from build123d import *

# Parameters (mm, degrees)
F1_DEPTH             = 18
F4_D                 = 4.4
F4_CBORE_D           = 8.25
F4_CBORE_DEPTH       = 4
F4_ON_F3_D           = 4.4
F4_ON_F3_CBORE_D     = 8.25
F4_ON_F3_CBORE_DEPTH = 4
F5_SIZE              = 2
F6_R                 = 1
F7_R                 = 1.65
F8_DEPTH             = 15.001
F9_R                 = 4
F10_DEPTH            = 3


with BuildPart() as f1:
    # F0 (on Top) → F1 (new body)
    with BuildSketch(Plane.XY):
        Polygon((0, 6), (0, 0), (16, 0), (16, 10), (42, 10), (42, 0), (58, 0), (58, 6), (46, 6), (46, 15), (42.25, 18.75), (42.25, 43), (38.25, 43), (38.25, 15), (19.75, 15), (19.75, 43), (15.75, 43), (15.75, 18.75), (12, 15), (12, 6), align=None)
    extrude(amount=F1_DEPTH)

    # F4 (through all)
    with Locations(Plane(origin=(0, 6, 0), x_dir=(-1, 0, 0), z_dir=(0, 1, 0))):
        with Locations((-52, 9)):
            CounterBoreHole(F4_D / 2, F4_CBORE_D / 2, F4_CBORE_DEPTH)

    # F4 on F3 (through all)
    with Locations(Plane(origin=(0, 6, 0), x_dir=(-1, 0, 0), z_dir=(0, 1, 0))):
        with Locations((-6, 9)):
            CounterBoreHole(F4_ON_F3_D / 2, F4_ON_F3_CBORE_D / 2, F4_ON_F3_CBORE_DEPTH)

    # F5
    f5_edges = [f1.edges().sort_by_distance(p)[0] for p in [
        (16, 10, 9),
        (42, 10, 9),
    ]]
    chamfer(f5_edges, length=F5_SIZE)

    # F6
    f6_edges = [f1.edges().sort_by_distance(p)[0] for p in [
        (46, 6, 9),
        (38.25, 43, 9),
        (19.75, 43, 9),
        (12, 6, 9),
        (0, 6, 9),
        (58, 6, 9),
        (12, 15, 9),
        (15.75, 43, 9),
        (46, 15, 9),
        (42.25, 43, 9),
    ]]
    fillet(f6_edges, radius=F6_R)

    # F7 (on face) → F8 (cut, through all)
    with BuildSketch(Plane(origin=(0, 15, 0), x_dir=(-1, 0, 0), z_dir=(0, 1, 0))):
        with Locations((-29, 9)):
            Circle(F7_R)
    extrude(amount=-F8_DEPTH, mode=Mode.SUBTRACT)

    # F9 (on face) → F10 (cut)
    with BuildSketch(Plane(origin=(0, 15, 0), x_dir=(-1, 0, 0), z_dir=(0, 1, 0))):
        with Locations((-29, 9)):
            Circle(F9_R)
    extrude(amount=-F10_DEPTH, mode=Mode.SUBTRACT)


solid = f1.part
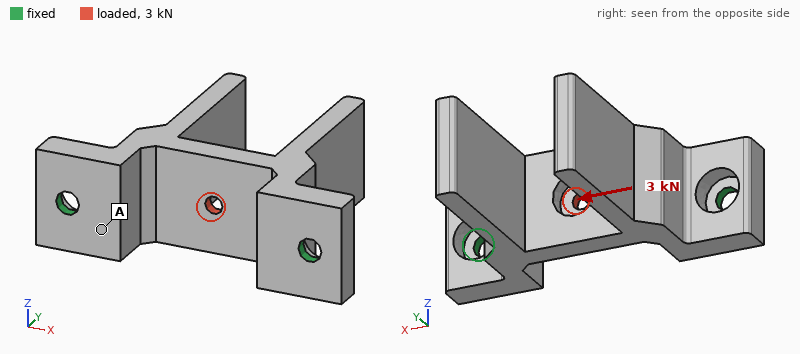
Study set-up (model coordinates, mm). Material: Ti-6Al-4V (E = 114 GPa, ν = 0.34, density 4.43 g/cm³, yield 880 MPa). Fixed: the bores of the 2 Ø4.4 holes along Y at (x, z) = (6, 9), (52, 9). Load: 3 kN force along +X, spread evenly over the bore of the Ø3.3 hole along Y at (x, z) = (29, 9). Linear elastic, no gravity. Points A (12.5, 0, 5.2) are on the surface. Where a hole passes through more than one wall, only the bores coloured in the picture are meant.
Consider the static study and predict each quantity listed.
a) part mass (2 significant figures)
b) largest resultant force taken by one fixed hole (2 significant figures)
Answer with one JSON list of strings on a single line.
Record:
["48 g", "1.6 kN"]
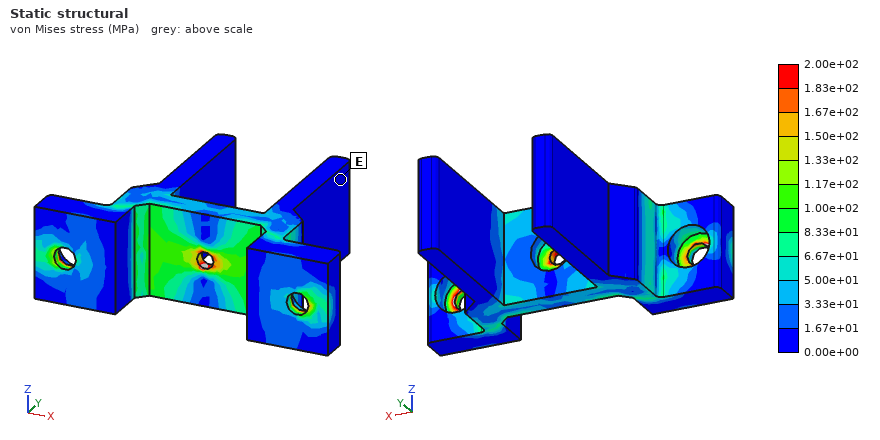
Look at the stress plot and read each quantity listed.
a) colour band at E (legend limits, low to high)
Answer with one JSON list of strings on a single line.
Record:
["0.00e+00 to 1.67e+01 MPa"]
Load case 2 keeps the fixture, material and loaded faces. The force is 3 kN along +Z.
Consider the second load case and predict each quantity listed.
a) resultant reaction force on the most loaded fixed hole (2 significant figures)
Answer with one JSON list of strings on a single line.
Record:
["1.5 kN"]
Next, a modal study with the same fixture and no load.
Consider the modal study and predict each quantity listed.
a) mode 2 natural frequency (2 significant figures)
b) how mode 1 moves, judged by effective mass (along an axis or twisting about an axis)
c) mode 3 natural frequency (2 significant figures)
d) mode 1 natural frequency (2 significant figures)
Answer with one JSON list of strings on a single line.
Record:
["3900 Hz", "along Z", "3900 Hz", "2100 Hz"]
